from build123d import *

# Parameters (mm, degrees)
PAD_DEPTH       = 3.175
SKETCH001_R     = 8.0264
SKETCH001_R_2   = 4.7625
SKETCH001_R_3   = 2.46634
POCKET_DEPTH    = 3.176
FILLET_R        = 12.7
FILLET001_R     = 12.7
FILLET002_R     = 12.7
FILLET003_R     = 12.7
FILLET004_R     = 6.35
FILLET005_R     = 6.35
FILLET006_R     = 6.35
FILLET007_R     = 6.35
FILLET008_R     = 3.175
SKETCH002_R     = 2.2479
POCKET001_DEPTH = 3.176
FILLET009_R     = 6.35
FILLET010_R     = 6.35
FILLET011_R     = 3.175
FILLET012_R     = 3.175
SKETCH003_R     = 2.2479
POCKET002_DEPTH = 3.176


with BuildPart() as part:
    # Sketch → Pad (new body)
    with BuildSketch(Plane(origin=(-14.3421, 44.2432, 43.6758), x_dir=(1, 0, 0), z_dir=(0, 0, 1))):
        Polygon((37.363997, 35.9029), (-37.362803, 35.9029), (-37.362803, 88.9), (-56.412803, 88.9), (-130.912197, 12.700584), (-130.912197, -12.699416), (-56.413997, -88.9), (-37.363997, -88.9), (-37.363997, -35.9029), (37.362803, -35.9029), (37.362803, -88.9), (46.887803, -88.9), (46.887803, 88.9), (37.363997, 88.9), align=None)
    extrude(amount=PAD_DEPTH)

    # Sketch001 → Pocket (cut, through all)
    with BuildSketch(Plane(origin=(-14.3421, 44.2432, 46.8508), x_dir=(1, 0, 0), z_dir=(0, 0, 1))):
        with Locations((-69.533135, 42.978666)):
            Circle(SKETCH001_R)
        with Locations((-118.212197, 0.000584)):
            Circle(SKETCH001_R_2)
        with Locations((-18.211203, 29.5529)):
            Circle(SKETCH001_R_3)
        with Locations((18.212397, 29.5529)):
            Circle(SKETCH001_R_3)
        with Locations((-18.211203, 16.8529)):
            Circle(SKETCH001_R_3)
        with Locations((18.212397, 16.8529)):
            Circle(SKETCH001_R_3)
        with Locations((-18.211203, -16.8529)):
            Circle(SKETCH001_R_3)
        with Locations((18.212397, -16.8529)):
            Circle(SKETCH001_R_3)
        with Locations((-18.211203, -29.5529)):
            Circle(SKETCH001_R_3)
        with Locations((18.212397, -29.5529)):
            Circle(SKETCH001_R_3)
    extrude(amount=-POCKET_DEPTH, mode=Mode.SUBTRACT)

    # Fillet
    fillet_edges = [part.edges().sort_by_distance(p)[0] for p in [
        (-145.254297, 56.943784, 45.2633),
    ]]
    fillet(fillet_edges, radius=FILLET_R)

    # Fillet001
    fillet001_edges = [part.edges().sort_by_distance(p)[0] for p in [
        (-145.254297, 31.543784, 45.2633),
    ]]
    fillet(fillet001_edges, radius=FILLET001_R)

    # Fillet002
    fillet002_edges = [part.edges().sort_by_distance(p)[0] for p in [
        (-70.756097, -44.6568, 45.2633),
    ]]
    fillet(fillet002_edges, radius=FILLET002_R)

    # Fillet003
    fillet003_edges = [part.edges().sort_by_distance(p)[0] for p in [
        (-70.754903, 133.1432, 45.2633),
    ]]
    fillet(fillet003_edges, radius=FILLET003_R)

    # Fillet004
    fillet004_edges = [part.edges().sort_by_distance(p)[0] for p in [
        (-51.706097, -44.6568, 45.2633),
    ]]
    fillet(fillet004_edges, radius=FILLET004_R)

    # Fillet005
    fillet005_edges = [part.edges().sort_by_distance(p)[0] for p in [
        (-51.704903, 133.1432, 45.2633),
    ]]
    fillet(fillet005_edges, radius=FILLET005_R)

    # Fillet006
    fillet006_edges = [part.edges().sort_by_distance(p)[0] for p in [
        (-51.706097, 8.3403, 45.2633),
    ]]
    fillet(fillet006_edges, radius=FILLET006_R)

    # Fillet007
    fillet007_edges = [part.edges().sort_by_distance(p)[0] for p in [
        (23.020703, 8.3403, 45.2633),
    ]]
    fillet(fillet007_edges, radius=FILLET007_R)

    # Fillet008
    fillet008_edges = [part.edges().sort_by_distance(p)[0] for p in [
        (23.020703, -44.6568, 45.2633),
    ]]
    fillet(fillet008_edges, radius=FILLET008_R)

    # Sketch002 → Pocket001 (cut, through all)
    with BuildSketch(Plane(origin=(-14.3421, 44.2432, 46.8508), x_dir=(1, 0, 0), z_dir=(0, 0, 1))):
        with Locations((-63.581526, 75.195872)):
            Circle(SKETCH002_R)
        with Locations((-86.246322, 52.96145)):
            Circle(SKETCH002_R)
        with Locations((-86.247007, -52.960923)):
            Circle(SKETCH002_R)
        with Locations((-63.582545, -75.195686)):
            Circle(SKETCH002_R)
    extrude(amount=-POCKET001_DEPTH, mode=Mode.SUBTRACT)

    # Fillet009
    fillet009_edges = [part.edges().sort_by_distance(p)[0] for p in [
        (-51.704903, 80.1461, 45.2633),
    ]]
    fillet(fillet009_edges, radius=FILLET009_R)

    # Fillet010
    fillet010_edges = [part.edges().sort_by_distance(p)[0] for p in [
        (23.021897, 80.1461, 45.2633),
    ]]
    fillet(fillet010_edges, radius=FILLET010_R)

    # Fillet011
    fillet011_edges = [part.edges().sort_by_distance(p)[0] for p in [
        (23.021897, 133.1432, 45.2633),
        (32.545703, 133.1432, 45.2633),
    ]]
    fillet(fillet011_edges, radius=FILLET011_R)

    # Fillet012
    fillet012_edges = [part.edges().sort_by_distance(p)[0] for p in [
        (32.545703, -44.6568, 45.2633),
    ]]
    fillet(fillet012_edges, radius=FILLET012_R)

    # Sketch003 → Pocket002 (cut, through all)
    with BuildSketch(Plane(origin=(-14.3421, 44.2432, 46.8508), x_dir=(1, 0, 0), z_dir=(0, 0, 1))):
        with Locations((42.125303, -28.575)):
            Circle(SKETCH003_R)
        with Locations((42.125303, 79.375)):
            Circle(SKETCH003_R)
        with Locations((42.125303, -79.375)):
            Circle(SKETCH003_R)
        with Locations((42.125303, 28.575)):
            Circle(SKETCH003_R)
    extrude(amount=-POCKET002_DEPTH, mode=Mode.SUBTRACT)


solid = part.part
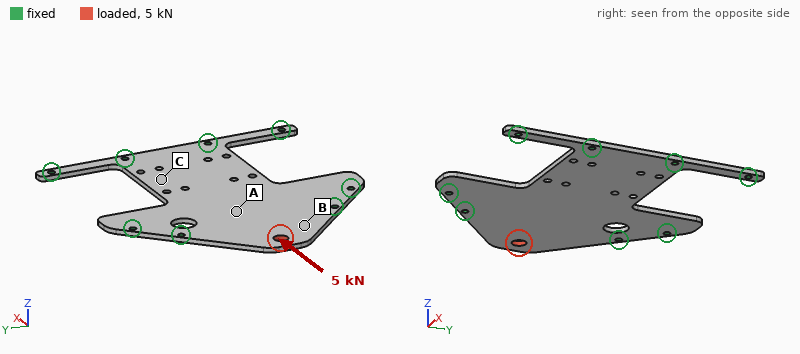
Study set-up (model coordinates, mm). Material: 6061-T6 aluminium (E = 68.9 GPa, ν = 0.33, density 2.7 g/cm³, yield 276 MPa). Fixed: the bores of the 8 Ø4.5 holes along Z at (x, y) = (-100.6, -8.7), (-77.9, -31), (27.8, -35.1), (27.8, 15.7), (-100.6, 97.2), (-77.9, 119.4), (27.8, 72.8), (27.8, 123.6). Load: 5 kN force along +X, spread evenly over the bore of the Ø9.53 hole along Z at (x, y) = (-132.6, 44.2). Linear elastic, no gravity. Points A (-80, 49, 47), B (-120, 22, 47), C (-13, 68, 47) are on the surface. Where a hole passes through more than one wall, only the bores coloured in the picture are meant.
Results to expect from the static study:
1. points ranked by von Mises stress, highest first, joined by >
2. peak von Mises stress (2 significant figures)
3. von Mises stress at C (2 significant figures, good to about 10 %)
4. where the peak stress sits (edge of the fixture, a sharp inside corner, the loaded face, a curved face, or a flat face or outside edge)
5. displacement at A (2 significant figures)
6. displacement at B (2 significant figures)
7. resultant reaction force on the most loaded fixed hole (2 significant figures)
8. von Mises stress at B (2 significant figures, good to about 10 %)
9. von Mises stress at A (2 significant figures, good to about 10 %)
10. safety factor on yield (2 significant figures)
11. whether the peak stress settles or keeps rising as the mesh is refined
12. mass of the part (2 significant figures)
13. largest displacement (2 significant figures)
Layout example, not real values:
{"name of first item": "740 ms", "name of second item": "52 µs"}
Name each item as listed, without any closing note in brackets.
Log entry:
{"points ranked by von Mises stress, highest first, joined by >": "B > A > C", "peak von Mises stress": "110 MPa", "von Mises stress at C": "7.6 MPa", "where the peak stress sits": "the loaded face", "displacement at A": "19 µm", "displacement at B": "22 µm", "resultant reaction force on the most loaded fixed hole": "1.6 kN", "von Mises stress at B": "25 MPa", "von Mises stress at A": "17 MPa", "safety factor on yield": "2.5", "whether the peak stress settles or keeps rising as the mesh is refined": "settles", "mass of the part": "150 g", "largest displacement": "48 µm"}
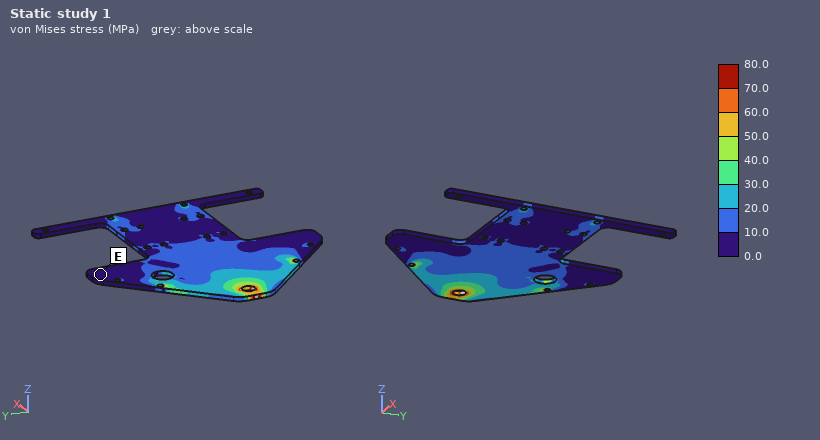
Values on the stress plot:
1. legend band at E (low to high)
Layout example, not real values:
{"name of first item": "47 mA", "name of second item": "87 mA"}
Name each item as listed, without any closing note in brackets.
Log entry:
{"legend band at E": "0.0 to 10.0 MPa"}
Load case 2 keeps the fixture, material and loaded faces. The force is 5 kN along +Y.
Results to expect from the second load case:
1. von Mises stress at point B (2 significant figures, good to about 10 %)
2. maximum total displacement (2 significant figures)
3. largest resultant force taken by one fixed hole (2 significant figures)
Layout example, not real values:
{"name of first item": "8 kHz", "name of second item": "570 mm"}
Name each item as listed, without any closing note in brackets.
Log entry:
{"von Mises stress at point B": "35 MPa", "maximum total displacement": "55 µm", "largest resultant force taken by one fixed hole": "2.5 kN"}
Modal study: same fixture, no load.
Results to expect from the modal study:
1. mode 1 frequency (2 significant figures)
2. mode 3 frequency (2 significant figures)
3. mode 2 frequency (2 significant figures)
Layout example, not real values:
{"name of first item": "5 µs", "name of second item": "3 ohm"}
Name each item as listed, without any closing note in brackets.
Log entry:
{"mode 1 frequency": "890 Hz", "mode 3 frequency": "1800 Hz", "mode 2 frequency": "920 Hz"}
